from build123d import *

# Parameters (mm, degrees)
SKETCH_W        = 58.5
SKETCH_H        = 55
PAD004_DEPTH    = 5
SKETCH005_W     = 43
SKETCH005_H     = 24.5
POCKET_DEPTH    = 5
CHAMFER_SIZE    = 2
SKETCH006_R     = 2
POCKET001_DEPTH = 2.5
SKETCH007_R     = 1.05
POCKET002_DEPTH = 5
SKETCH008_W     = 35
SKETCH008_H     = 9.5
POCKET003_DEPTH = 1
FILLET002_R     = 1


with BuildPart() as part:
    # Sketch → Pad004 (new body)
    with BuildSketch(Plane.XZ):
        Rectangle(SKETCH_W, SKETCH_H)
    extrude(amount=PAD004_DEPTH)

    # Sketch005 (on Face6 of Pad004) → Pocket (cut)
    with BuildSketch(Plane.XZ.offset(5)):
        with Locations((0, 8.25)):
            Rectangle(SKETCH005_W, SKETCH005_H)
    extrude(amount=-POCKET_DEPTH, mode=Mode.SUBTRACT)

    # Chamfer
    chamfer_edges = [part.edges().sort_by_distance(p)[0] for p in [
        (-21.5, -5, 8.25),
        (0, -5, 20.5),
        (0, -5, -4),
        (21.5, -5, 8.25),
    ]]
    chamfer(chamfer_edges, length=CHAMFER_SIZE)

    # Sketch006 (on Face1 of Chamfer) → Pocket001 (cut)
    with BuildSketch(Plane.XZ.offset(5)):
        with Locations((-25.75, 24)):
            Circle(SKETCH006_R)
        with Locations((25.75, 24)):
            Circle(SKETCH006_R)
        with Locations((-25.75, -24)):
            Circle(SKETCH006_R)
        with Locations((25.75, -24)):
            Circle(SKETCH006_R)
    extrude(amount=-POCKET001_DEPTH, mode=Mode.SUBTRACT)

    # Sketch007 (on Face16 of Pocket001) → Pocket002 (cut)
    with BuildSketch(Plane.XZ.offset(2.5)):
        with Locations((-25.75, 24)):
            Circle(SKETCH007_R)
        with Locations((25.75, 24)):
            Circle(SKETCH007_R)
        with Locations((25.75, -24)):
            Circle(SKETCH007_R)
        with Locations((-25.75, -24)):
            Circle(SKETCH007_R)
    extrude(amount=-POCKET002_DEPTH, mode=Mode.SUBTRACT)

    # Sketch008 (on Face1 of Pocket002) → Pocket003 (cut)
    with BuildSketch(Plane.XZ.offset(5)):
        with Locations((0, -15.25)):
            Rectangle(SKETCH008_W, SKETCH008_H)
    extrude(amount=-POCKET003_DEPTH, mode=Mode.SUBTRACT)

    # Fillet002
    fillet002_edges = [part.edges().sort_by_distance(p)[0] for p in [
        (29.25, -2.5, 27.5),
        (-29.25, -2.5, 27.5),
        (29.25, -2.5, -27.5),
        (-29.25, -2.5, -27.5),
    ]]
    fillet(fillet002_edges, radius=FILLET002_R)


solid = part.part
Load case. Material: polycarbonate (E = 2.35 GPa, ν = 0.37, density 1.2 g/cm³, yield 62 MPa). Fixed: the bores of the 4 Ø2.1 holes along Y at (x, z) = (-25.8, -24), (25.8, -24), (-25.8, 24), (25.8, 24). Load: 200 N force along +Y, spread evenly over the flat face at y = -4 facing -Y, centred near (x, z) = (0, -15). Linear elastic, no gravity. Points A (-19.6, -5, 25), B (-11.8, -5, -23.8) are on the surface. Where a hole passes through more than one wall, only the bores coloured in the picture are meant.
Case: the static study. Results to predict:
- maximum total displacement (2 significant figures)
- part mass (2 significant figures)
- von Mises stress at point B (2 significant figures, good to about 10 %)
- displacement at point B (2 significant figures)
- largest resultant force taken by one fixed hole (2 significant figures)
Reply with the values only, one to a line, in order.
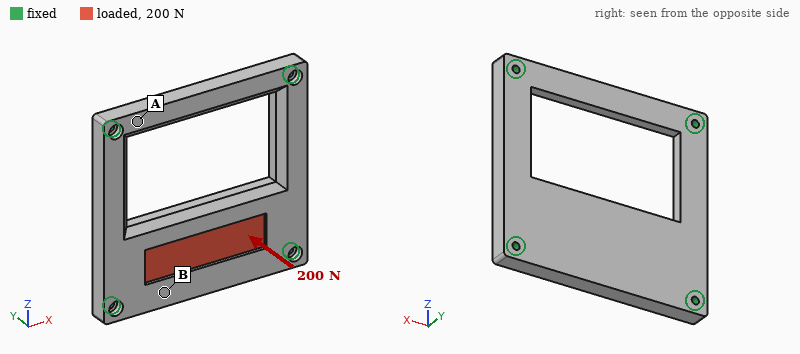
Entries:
0.78 mm
12 g
8.5 MPa
0.33 mm
120 N
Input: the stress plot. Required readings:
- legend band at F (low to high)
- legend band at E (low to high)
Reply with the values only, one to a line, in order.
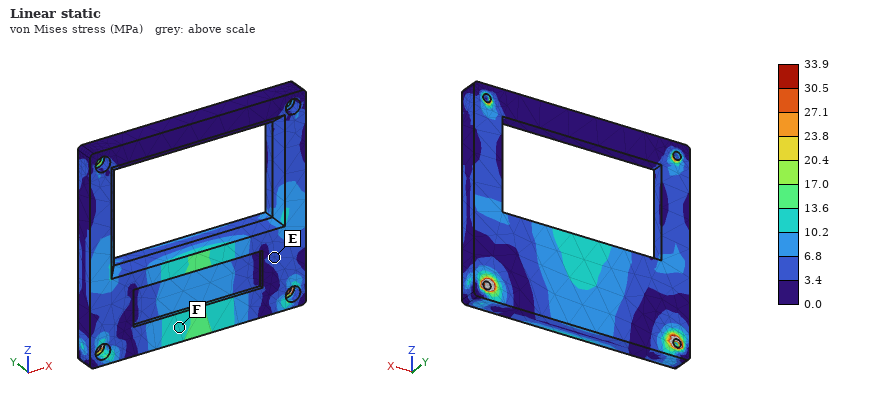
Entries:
10.2 to 13.6 MPa
3.4 to 6.8 MPa
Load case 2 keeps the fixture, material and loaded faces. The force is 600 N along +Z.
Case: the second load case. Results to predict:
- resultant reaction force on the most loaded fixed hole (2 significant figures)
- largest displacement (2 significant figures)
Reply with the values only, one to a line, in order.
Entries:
270 N
0.39 mm
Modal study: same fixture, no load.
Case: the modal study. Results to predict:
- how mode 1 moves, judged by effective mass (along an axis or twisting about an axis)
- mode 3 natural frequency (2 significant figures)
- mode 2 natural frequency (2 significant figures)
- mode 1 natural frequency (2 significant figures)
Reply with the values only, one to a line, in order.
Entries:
along Y
2300 Hz
2100 Hz
1300 Hz
